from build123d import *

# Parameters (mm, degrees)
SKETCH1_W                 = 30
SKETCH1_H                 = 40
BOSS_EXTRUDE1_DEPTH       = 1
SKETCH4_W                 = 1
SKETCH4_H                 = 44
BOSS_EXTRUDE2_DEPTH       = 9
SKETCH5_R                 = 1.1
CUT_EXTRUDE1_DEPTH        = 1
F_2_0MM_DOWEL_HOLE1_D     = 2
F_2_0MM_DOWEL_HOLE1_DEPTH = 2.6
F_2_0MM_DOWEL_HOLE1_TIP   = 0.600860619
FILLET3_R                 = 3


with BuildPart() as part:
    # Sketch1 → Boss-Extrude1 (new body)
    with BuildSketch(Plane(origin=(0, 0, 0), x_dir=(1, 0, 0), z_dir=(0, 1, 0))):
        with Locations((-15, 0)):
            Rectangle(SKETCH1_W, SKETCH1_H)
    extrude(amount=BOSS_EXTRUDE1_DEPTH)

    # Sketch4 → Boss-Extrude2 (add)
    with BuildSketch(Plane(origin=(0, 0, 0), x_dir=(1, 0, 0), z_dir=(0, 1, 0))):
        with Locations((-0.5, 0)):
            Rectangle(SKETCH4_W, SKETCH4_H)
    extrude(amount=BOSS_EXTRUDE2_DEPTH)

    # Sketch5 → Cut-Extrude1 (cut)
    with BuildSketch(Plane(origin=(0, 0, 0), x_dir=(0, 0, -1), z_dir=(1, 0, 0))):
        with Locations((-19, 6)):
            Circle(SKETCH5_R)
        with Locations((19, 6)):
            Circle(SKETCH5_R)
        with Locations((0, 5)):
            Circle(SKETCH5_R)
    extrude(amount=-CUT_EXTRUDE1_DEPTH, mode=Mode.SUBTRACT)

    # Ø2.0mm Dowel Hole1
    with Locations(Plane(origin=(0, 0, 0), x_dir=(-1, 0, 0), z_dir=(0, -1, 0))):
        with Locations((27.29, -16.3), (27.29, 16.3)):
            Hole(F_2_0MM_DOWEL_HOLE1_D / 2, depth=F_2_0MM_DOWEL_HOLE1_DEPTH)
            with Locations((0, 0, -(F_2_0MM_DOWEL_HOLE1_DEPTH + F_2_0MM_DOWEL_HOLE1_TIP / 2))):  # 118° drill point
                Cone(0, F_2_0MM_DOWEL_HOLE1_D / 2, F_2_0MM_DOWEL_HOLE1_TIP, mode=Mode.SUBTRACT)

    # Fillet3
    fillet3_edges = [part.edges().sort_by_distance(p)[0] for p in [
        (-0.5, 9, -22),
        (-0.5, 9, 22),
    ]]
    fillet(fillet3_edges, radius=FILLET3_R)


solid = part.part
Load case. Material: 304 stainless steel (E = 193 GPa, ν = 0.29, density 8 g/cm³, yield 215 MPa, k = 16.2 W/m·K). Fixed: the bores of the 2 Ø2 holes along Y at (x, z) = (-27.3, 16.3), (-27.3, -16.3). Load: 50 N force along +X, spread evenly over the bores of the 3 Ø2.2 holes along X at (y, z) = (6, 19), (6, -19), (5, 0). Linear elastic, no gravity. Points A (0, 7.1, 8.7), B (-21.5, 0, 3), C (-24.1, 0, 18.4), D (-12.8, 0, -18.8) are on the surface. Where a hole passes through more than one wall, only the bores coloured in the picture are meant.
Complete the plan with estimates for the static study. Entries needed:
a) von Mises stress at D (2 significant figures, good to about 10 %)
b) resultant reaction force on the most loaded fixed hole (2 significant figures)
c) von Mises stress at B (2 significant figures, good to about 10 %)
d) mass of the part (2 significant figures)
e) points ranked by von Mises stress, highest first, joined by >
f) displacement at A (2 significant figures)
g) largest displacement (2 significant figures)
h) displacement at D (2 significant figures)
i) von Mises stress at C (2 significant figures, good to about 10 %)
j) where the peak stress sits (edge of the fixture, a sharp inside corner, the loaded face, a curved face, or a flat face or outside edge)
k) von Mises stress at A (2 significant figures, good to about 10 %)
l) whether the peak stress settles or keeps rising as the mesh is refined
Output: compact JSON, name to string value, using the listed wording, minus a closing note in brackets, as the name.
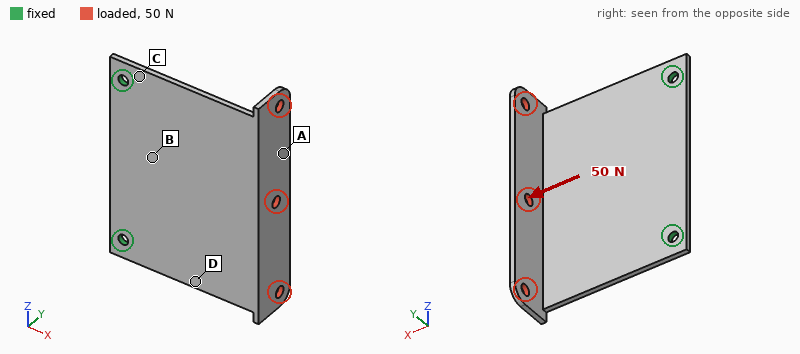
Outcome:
{"von Mises stress at D": "40 MPa", "resultant reaction force on the most loaded fixed hole": "26 N", "von Mises stress at B": "25 MPa", "mass of the part": "12 g", "points ranked by von Mises stress, highest first, joined by >": "C > D > B > A", "displacement at A": "0.20 mm", "largest displacement": "0.22 mm", "displacement at D": "0.055 mm", "von Mises stress at C": "61 MPa", "where the peak stress sits": "edge of the fixture", "von Mises stress at A": "15 MPa", "whether the peak stress settles or keeps rising as the mesh is refined": "keeps rising"}
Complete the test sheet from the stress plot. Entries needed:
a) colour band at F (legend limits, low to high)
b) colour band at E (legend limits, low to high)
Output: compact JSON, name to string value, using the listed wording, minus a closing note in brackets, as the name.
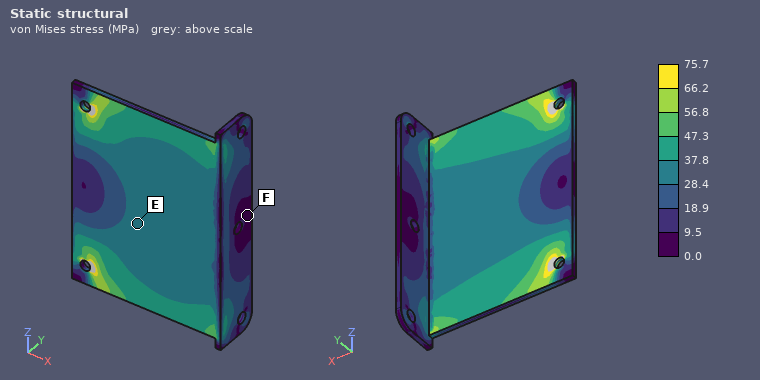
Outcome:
{"colour band at F": "0.0 to 9.5 MPa", "colour band at E": "28.4 to 37.8 MPa"}
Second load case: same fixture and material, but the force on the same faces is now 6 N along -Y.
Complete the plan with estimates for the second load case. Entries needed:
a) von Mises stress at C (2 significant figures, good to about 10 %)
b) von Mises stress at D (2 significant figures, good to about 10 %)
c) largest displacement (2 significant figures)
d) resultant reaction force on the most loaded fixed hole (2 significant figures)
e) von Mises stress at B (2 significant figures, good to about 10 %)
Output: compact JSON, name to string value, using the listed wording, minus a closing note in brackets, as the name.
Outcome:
{"von Mises stress at C": "37 MPa", "von Mises stress at D": "13 MPa", "largest displacement": "90 µm", "resultant reaction force on the most loaded fixed hole": "3.0 N", "von Mises stress at B": "11 MPa"}
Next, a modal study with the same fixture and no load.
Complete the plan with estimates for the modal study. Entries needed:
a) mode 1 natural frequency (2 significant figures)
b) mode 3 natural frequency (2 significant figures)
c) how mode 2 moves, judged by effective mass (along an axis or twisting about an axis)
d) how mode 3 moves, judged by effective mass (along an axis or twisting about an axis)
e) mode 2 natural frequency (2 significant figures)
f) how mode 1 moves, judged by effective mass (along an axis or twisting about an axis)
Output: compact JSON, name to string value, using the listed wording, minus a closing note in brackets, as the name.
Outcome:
{"mode 1 natural frequency": "600 Hz", "mode 3 natural frequency": "3600 Hz", "how mode 2 moves, judged by effective mass": "twisting about X", "how mode 3 moves, judged by effective mass": "along Y", "mode 2 natural frequency": "1400 Hz", "how mode 1 moves, judged by effective mass": "along Y"}
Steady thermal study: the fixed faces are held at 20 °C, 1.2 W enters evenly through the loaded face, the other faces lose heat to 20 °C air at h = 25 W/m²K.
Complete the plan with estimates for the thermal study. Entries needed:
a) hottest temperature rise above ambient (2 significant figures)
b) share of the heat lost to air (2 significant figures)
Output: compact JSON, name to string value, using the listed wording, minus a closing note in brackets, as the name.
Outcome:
{"hottest temperature rise above ambient": "37 K", "share of the heat lost to air": "82 %"}
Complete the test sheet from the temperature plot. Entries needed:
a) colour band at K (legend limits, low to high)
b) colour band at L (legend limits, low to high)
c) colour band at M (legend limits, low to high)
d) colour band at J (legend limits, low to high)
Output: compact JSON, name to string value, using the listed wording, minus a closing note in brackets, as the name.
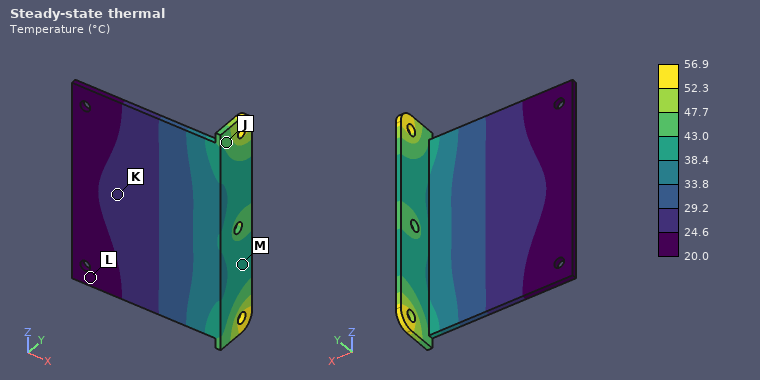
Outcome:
{"colour band at K": "24.6 to 29.2 °C", "colour band at L": "20.0 to 24.6 °C", "colour band at M": "38.4 to 43.0 °C", "colour band at J": "43.0 to 47.7 °C"}
